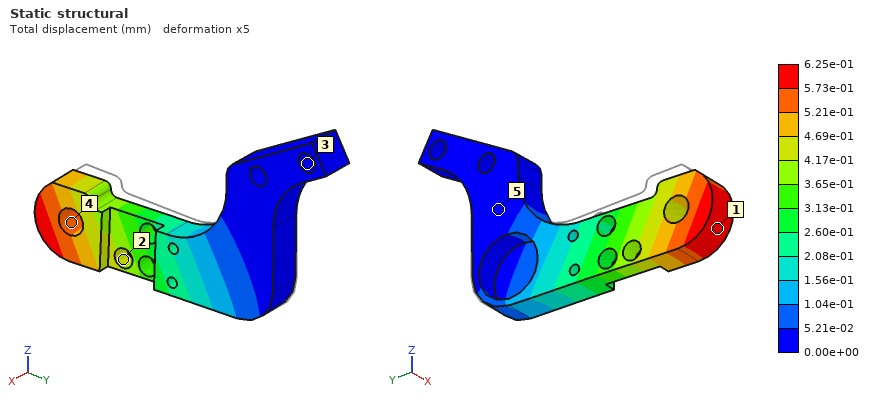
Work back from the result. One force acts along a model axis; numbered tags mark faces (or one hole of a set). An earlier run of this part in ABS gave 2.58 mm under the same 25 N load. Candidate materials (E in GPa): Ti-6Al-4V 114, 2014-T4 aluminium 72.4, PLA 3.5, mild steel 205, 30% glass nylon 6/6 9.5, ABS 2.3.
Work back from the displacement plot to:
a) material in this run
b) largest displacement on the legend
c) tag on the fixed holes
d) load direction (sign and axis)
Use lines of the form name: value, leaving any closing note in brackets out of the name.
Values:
material in this run: 30% glass nylon 6/6
largest displacement on the legend: 6.25e-01 mm
tag on the fixed holes: 3
load direction: +X
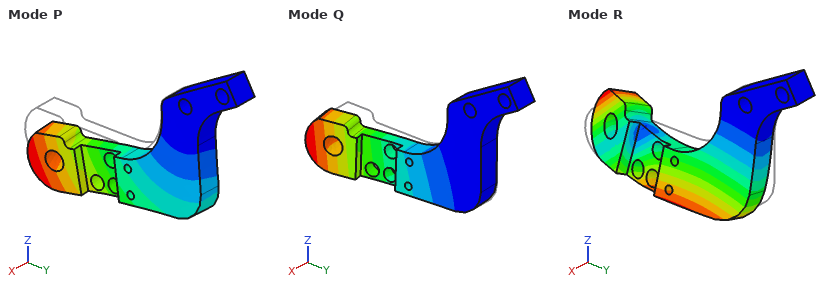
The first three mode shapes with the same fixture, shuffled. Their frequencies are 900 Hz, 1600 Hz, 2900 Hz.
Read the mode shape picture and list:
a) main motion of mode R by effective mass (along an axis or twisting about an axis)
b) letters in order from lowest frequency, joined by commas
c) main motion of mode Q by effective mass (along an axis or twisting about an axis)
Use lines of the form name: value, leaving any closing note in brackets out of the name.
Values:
main motion of mode R by effective mass: along X
letters in order from lowest frequency, joined by commas: Q, P, R
main motion of mode Q by effective mass: along X
